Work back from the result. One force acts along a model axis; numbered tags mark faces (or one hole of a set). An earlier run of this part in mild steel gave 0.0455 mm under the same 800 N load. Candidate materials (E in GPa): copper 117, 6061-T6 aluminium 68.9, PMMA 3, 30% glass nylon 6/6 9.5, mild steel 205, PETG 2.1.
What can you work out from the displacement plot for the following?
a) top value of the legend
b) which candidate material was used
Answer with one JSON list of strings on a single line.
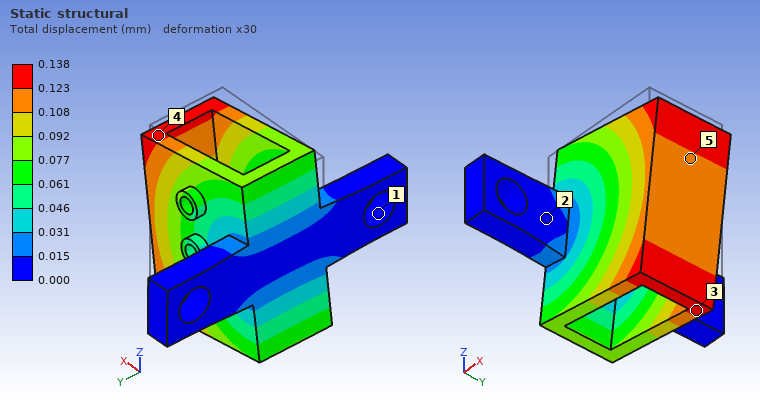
["0.138 mm", "6061-T6 aluminium"]
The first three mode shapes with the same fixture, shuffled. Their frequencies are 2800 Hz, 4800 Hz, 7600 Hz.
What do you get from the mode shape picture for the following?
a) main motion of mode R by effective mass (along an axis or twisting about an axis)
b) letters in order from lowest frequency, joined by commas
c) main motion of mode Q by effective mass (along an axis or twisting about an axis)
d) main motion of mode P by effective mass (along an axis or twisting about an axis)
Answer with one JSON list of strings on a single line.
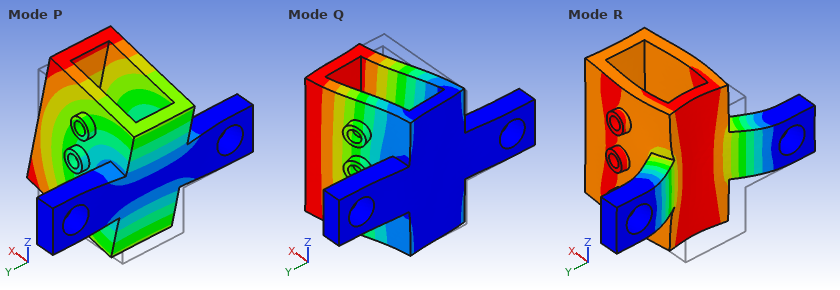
["along X", "P, Q, R", "along Y", "along Z"]
